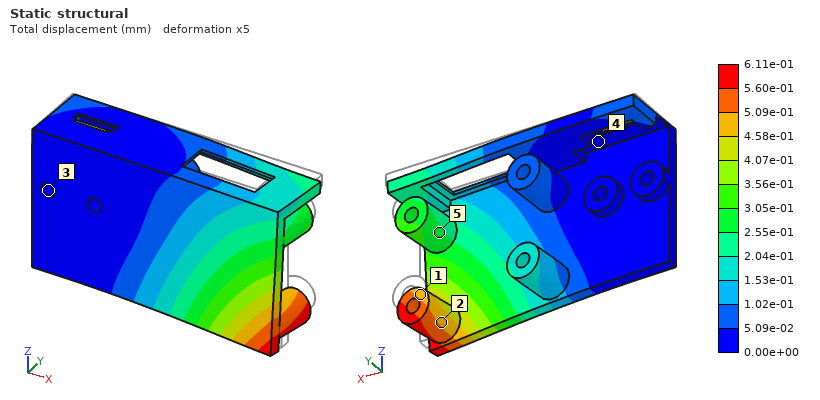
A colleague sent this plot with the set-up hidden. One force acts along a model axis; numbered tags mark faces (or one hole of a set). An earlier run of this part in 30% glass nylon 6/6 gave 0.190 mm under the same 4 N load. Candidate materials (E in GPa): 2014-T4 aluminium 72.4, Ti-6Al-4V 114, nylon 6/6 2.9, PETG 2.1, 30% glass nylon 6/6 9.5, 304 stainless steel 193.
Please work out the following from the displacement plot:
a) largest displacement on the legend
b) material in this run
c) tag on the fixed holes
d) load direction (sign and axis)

6.11e-01 mm
nylon 6/6
3
-Y
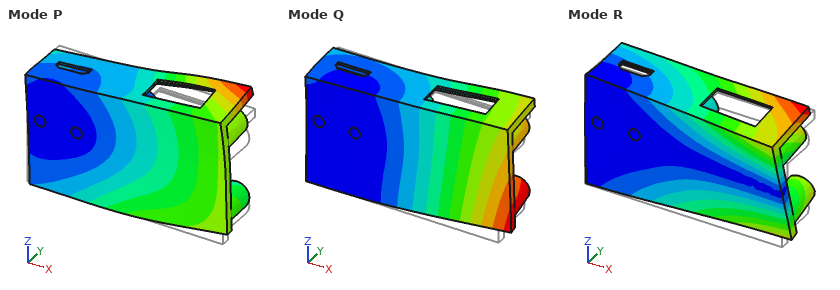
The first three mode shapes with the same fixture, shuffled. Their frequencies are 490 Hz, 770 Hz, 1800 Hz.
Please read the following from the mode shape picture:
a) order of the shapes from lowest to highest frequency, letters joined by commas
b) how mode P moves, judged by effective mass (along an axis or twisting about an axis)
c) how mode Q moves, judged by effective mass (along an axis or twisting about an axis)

Q, R, P
along Z
along Y
